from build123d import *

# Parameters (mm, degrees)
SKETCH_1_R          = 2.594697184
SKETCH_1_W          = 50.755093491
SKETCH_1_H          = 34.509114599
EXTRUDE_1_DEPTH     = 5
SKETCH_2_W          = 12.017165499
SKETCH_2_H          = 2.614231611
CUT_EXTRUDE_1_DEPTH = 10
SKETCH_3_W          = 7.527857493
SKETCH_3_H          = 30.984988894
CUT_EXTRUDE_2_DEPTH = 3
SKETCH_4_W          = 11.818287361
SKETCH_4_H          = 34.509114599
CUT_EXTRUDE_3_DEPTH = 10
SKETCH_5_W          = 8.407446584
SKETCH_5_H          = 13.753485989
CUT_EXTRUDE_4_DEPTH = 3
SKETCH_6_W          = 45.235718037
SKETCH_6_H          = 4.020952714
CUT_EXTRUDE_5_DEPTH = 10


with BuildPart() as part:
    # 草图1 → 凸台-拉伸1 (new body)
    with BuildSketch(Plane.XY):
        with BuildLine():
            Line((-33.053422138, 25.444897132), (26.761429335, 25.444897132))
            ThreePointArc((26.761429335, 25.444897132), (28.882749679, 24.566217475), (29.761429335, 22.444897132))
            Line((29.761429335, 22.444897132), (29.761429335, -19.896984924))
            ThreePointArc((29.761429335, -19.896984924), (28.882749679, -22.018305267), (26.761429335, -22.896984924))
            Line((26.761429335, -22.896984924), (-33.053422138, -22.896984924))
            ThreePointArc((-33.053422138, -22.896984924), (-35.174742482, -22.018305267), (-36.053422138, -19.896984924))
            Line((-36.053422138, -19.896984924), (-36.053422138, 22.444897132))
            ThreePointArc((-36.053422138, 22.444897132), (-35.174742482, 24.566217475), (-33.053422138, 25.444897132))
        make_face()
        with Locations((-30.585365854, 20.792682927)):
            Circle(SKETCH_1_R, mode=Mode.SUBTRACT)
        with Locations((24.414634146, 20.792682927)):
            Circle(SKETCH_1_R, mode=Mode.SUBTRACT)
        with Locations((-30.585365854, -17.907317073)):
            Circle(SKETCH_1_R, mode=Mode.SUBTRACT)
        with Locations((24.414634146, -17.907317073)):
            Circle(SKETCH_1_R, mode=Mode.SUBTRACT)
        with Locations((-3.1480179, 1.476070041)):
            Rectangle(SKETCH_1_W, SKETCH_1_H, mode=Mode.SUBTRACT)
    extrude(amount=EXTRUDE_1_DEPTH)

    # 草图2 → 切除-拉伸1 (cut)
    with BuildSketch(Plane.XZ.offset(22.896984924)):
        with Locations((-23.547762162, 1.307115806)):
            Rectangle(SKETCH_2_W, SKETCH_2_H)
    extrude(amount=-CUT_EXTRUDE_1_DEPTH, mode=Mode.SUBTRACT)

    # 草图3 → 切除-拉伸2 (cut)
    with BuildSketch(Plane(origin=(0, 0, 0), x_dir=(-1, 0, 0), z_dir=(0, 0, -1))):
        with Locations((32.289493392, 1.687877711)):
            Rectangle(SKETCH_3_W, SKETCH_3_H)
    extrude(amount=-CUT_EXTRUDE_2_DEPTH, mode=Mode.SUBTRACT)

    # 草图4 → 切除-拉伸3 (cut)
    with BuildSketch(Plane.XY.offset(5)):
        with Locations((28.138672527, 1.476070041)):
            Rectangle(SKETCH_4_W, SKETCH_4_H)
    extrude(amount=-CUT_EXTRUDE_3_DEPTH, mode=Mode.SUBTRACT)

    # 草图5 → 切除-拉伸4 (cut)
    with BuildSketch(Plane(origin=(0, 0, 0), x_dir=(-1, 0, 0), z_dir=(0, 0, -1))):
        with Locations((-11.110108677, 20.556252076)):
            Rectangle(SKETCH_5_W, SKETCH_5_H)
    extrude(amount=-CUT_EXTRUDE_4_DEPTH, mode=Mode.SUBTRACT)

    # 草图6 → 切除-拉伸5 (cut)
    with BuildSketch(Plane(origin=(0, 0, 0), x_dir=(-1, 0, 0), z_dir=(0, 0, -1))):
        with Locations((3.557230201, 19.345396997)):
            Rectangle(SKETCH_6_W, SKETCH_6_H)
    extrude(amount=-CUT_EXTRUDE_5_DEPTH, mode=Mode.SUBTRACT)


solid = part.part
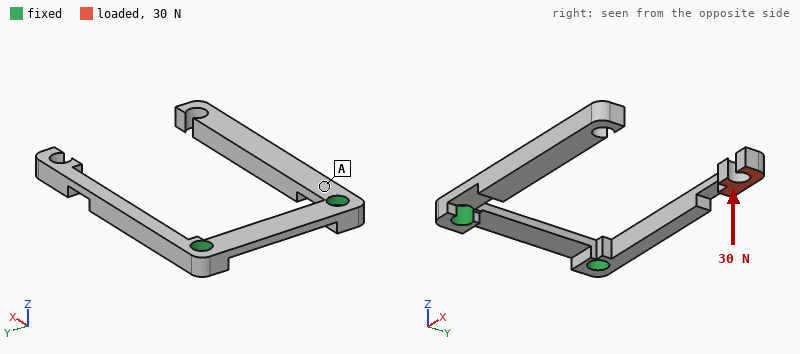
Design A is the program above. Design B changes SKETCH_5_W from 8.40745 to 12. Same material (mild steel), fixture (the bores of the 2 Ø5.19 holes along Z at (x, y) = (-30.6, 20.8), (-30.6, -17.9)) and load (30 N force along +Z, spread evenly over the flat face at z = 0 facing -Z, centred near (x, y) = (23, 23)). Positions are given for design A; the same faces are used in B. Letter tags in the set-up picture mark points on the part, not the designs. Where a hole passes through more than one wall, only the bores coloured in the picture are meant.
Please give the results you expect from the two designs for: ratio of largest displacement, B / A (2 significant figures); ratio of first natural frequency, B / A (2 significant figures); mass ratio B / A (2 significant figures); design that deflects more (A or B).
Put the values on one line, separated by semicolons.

1.2; 1.0; 0.99; B
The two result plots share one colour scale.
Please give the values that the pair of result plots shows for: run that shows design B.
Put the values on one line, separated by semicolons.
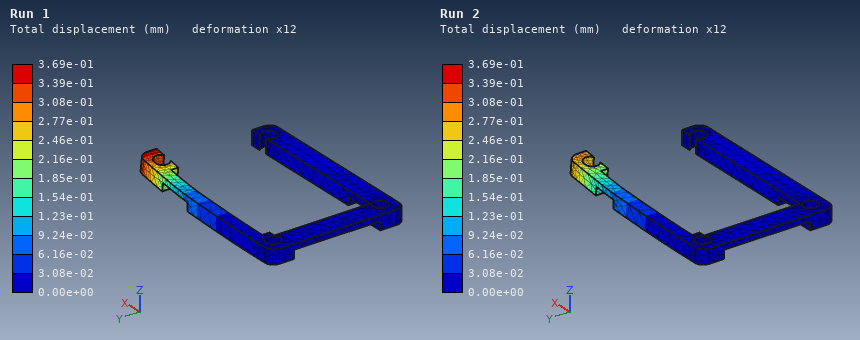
Run 1
